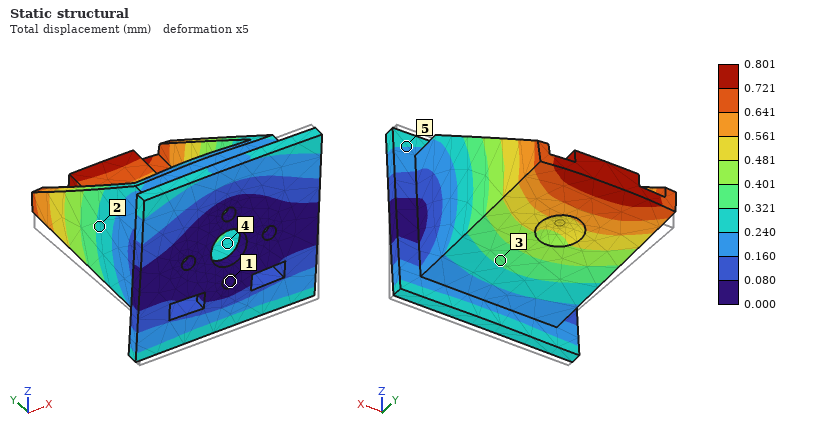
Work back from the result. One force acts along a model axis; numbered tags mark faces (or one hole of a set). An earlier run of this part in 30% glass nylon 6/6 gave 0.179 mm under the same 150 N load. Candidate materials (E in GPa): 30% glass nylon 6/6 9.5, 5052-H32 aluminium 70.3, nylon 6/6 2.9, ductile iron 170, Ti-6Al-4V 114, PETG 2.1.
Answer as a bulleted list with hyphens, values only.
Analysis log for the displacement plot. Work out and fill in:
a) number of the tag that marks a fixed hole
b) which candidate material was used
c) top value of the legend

- 1
- PETG
- 0.801 mm
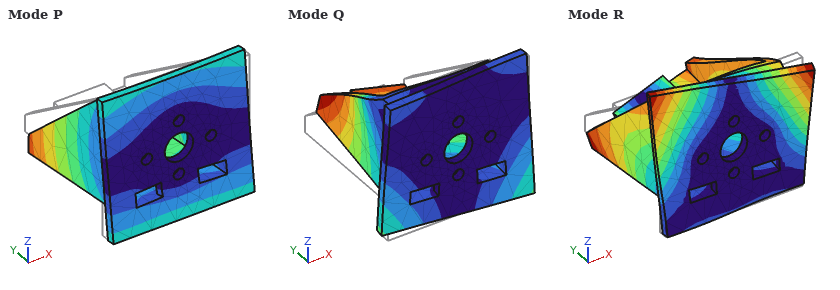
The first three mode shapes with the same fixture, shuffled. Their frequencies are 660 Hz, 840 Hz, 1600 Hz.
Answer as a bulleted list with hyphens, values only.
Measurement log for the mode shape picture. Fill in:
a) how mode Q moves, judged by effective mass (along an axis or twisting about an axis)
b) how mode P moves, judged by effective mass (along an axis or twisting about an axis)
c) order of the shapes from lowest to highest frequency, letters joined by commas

- along X
- along Z
- Q, P, R
